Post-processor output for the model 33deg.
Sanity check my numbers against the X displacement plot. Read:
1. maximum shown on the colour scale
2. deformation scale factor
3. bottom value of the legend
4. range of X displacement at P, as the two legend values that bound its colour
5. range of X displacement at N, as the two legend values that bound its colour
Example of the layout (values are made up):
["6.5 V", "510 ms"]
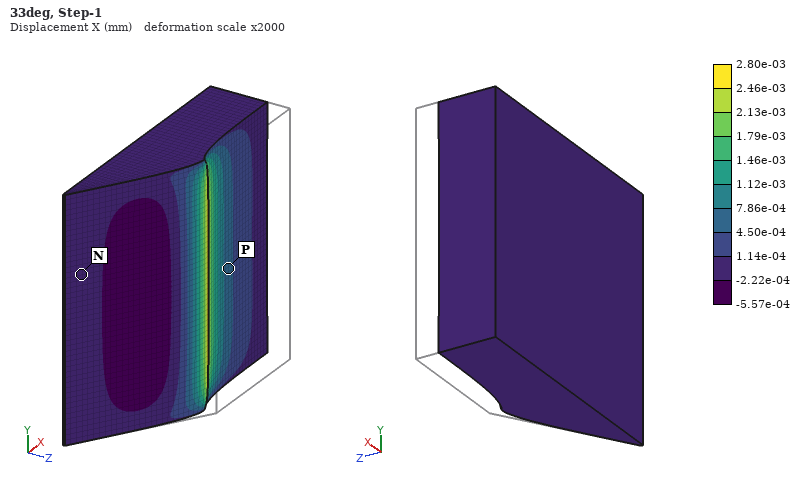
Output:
["2.80e-03 mm", "2000", "-5.57e-04 mm", "4.50e-04 to 7.86e-04 mm", "-2.22e-04 to 1.14e-04 mm"]
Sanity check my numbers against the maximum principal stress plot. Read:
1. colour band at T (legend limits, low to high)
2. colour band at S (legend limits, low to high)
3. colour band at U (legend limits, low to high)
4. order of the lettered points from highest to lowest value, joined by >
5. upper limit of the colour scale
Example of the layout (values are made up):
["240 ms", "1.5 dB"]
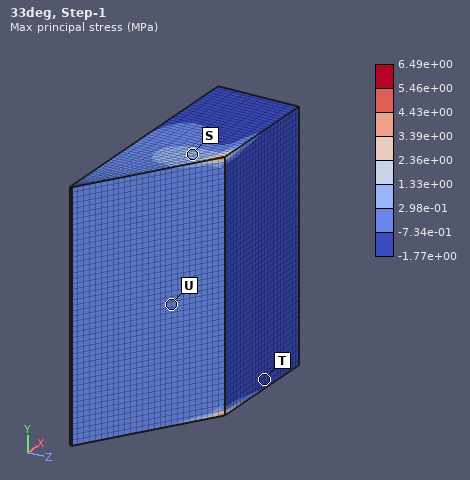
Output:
["-1.77e+00 to -7.34e-01 MPa", "2.98e-01 to 1.33e+00 MPa", "-7.34e-01 to 2.98e-01 MPa", "S > U > T", "6.49e+00 MPa"]
